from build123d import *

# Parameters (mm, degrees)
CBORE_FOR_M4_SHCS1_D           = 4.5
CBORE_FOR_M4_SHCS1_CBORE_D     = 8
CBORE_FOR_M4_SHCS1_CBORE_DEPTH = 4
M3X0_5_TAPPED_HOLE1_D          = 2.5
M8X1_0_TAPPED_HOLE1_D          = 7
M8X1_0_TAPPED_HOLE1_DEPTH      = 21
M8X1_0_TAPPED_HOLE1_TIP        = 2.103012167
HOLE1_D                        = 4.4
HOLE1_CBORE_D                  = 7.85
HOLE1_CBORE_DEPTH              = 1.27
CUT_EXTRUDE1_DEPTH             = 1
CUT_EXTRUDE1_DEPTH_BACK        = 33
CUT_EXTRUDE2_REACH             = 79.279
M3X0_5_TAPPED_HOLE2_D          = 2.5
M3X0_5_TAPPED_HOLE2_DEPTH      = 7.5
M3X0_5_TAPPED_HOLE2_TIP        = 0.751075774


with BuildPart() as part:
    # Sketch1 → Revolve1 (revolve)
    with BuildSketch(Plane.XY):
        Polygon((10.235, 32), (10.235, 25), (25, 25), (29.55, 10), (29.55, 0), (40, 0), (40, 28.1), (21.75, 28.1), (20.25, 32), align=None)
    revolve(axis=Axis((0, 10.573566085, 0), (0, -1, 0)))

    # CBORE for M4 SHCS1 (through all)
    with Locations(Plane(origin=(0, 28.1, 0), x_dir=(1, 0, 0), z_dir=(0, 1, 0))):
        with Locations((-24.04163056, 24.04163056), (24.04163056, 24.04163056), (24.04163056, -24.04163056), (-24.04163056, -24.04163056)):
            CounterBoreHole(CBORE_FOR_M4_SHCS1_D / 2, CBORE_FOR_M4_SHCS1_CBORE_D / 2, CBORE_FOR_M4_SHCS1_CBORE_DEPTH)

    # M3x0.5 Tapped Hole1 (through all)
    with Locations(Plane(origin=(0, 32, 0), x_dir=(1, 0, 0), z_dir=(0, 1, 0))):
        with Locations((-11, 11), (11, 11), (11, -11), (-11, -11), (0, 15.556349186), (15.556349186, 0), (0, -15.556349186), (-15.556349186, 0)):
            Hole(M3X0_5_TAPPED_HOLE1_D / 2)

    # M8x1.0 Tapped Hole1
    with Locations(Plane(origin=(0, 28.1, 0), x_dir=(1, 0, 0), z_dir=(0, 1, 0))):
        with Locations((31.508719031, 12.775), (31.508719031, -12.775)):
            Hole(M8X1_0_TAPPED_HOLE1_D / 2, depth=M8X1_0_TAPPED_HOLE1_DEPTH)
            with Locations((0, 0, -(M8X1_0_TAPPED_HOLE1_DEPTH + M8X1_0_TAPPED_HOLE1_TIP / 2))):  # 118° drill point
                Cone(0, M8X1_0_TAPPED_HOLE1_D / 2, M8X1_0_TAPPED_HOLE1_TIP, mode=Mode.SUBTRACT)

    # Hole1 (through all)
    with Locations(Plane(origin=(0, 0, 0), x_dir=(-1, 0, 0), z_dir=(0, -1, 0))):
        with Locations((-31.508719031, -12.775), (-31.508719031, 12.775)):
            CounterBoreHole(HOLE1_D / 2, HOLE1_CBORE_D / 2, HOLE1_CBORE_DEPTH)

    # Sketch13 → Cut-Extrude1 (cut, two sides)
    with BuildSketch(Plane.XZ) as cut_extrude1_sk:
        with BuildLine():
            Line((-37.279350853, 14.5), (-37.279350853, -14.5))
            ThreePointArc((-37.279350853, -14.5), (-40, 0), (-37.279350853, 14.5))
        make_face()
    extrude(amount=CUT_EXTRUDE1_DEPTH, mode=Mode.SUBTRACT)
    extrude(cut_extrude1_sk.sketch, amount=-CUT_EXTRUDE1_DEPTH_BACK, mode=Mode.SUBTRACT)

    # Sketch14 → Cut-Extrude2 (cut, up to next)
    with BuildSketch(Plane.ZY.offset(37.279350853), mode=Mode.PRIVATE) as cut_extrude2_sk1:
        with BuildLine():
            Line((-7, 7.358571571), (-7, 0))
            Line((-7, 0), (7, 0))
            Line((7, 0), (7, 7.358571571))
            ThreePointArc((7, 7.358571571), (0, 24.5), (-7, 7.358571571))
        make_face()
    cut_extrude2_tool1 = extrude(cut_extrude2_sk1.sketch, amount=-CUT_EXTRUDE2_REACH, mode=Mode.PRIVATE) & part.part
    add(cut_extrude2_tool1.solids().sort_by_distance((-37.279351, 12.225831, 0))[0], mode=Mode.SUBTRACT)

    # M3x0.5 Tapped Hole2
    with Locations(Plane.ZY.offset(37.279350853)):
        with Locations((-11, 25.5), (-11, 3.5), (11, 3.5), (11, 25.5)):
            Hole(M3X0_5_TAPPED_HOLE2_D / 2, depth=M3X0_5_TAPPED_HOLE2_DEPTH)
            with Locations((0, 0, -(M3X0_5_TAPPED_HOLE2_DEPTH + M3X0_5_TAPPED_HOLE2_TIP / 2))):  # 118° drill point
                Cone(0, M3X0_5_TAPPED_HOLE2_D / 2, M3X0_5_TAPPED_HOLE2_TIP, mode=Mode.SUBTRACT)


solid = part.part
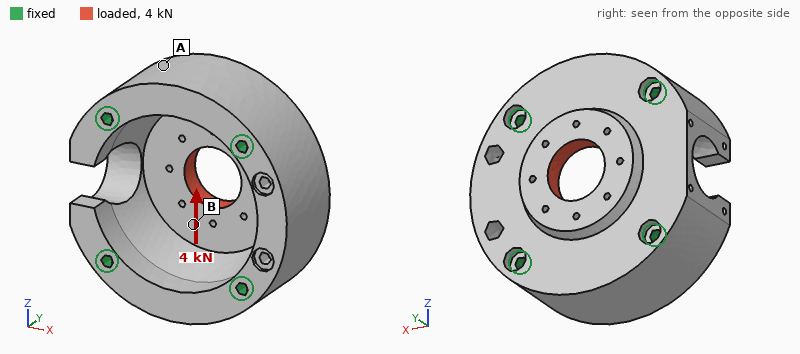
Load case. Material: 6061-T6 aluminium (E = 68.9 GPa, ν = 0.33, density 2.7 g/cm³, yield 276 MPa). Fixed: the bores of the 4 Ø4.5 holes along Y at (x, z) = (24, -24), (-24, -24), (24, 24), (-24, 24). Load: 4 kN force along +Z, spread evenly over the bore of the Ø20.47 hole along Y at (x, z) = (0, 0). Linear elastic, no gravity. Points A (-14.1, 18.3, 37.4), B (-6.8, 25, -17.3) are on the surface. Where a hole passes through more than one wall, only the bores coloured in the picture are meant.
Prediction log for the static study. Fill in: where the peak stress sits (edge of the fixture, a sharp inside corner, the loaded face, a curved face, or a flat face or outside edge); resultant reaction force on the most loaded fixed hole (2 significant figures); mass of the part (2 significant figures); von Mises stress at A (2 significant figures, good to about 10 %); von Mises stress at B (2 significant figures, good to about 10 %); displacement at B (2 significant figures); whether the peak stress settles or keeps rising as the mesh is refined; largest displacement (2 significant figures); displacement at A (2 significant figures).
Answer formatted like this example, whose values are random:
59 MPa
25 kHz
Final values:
edge of the fixture
1.0 kN
190 g
4.0 MPa
12 MPa
5.1 µm
keeps rising
7.9 µm
1.9 µm
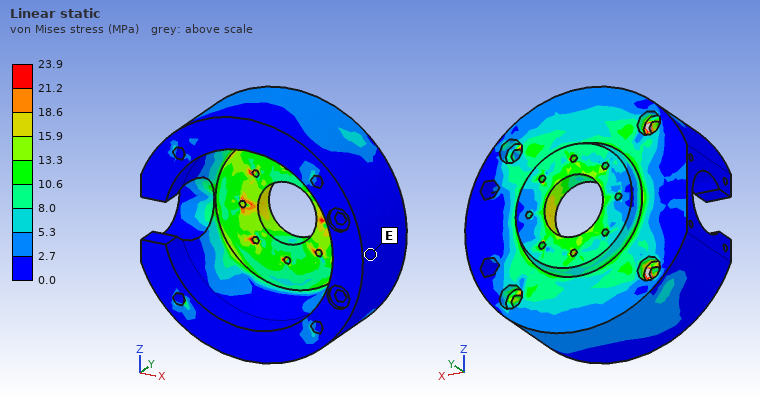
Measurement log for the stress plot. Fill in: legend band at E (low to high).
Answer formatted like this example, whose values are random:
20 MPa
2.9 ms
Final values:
0.0 to 2.7 MPa
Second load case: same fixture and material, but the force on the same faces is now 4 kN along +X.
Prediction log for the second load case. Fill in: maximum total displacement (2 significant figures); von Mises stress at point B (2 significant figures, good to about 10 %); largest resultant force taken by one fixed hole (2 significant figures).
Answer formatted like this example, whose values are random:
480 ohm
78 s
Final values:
8.2 µm
13 MPa
1.1 kN
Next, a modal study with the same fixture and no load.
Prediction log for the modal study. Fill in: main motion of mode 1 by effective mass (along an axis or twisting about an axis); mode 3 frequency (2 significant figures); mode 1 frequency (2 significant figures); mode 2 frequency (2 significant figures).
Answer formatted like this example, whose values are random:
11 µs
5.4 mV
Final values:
along Y
21 kHz
15 kHz
20 kHz
